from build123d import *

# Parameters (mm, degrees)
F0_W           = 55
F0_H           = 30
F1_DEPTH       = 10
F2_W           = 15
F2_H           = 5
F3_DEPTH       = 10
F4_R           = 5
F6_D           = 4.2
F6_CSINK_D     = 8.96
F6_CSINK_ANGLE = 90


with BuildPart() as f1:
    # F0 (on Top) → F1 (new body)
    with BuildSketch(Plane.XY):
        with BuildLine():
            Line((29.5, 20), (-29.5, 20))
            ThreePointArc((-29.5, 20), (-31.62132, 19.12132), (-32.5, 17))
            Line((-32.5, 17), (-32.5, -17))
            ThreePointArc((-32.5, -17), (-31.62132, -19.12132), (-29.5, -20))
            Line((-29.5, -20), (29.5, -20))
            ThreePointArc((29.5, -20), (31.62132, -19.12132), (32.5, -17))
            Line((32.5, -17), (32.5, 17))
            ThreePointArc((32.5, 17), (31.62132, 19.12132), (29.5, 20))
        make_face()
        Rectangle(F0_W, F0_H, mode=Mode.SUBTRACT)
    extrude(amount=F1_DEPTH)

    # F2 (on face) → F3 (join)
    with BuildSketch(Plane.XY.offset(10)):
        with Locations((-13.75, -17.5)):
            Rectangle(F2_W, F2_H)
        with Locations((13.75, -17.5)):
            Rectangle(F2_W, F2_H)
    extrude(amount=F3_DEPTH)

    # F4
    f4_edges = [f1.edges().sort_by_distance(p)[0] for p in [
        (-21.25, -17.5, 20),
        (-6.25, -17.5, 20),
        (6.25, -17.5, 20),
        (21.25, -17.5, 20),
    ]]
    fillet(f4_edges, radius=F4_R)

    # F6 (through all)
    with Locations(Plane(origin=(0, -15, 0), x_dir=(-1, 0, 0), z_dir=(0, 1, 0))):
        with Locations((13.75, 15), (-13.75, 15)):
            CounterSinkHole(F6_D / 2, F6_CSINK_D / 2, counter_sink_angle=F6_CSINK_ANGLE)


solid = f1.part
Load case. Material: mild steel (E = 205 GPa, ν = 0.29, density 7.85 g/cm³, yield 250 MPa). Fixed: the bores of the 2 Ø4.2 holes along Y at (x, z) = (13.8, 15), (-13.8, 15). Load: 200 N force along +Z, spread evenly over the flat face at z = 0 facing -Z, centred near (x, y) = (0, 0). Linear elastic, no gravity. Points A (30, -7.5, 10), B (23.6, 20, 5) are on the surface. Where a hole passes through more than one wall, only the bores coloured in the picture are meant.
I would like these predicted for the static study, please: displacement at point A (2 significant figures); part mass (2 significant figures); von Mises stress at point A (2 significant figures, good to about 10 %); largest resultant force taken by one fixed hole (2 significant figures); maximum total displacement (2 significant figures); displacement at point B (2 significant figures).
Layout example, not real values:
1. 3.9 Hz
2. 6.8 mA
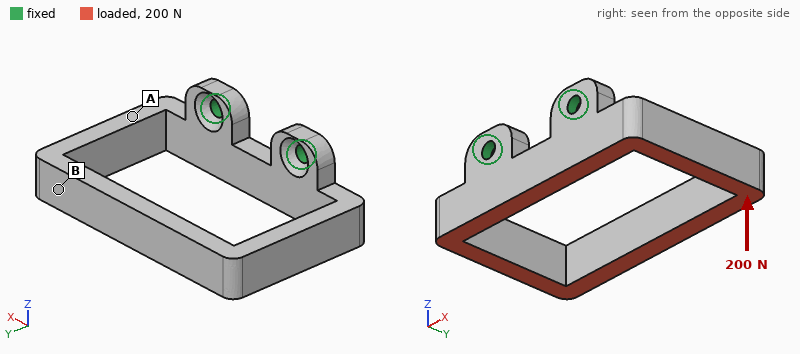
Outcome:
1. 17 µm
2. 83 g
3. 14 MPa
4. 130 N
5. 69 µm
6. 67 µm
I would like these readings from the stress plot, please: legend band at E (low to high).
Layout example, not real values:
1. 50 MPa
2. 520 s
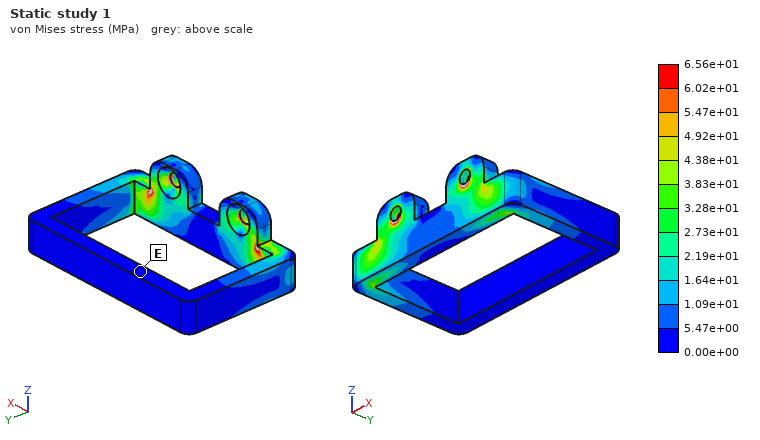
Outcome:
1. 0.00e+00 to 5.47e+00 MPa
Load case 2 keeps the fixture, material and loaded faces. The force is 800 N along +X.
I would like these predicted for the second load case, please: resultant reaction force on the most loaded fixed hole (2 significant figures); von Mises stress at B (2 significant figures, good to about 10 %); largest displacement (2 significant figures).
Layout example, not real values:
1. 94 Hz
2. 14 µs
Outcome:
1. 600 N
2. 63 MPa
3. 0.16 mm
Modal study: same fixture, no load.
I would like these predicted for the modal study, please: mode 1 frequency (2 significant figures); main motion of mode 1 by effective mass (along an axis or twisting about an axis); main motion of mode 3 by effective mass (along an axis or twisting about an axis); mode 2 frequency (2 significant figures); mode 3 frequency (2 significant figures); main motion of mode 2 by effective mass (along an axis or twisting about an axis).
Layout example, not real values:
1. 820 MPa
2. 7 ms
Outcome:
1. 1100 Hz
2. along Z
3. twisting about Y
4. 1400 Hz
5. 2500 Hz
6. along X
